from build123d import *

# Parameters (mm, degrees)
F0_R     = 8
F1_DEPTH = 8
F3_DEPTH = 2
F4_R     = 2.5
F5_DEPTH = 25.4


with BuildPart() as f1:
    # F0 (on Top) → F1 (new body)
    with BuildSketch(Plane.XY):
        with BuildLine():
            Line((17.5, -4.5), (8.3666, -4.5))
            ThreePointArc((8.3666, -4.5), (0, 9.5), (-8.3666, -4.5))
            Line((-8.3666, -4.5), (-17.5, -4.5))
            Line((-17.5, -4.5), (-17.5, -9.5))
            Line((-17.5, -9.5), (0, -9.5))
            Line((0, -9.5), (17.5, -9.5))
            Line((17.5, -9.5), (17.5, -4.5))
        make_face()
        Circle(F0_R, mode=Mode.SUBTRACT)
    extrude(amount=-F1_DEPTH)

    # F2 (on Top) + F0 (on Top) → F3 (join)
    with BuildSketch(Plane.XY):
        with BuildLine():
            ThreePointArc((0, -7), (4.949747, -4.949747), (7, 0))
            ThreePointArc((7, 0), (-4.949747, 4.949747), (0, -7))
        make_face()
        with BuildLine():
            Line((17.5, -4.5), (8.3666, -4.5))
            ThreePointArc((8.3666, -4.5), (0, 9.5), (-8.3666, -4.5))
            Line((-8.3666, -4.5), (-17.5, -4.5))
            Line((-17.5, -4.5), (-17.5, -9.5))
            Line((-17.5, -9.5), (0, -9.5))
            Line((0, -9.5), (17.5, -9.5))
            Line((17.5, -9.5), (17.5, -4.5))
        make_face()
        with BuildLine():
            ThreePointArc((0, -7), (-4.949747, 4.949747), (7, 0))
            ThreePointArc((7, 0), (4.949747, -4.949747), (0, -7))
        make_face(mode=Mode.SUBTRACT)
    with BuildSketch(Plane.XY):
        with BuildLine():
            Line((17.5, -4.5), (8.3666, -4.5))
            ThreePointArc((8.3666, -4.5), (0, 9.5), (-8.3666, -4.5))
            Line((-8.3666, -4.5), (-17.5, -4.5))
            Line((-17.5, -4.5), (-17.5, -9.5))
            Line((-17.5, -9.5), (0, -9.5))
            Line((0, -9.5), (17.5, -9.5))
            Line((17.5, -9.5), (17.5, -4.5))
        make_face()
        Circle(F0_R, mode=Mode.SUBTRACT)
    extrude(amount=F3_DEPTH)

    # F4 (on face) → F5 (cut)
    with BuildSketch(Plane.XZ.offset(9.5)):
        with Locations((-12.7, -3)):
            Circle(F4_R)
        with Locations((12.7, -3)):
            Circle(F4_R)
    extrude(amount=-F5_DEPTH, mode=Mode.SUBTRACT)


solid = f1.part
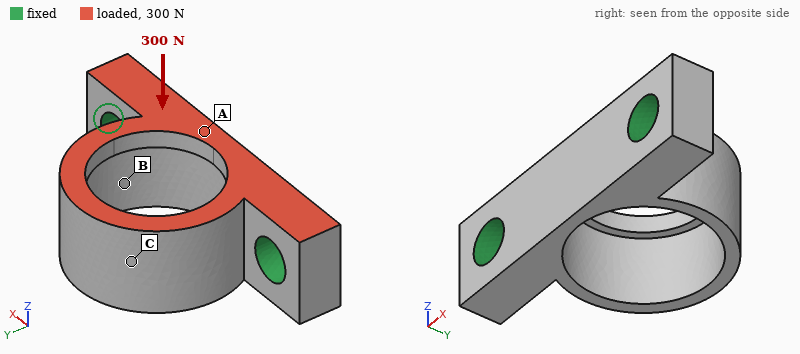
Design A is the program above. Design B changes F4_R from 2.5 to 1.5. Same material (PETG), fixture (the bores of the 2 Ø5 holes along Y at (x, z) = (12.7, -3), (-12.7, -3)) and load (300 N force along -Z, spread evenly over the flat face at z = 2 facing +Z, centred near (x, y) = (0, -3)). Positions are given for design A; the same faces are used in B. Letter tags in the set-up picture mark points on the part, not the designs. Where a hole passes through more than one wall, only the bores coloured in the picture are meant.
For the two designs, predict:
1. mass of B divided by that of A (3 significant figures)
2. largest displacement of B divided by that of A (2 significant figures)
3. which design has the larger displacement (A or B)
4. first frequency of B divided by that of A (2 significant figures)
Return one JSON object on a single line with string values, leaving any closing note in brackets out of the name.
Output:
{"mass of B divided by that of A": "1.07", "largest displacement of B divided by that of A": "1.2", "which design has the larger displacement": "B", "first frequency of B divided by that of A": "0.99"}
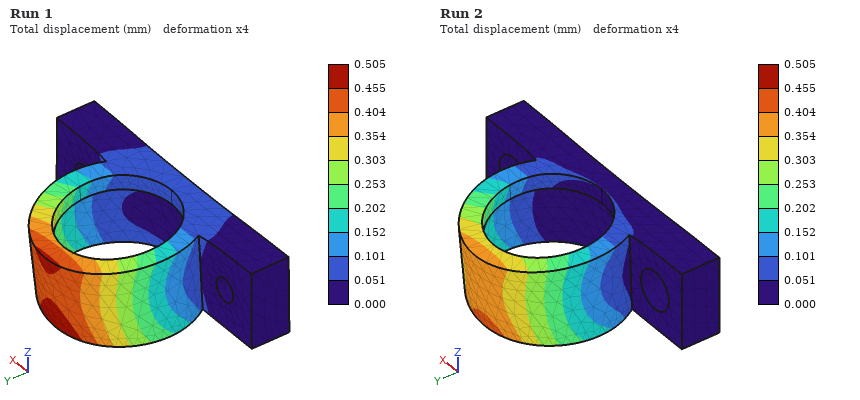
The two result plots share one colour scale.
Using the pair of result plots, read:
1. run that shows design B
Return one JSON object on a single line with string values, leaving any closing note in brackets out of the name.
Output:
{"run that shows design B": "Run 1"}
